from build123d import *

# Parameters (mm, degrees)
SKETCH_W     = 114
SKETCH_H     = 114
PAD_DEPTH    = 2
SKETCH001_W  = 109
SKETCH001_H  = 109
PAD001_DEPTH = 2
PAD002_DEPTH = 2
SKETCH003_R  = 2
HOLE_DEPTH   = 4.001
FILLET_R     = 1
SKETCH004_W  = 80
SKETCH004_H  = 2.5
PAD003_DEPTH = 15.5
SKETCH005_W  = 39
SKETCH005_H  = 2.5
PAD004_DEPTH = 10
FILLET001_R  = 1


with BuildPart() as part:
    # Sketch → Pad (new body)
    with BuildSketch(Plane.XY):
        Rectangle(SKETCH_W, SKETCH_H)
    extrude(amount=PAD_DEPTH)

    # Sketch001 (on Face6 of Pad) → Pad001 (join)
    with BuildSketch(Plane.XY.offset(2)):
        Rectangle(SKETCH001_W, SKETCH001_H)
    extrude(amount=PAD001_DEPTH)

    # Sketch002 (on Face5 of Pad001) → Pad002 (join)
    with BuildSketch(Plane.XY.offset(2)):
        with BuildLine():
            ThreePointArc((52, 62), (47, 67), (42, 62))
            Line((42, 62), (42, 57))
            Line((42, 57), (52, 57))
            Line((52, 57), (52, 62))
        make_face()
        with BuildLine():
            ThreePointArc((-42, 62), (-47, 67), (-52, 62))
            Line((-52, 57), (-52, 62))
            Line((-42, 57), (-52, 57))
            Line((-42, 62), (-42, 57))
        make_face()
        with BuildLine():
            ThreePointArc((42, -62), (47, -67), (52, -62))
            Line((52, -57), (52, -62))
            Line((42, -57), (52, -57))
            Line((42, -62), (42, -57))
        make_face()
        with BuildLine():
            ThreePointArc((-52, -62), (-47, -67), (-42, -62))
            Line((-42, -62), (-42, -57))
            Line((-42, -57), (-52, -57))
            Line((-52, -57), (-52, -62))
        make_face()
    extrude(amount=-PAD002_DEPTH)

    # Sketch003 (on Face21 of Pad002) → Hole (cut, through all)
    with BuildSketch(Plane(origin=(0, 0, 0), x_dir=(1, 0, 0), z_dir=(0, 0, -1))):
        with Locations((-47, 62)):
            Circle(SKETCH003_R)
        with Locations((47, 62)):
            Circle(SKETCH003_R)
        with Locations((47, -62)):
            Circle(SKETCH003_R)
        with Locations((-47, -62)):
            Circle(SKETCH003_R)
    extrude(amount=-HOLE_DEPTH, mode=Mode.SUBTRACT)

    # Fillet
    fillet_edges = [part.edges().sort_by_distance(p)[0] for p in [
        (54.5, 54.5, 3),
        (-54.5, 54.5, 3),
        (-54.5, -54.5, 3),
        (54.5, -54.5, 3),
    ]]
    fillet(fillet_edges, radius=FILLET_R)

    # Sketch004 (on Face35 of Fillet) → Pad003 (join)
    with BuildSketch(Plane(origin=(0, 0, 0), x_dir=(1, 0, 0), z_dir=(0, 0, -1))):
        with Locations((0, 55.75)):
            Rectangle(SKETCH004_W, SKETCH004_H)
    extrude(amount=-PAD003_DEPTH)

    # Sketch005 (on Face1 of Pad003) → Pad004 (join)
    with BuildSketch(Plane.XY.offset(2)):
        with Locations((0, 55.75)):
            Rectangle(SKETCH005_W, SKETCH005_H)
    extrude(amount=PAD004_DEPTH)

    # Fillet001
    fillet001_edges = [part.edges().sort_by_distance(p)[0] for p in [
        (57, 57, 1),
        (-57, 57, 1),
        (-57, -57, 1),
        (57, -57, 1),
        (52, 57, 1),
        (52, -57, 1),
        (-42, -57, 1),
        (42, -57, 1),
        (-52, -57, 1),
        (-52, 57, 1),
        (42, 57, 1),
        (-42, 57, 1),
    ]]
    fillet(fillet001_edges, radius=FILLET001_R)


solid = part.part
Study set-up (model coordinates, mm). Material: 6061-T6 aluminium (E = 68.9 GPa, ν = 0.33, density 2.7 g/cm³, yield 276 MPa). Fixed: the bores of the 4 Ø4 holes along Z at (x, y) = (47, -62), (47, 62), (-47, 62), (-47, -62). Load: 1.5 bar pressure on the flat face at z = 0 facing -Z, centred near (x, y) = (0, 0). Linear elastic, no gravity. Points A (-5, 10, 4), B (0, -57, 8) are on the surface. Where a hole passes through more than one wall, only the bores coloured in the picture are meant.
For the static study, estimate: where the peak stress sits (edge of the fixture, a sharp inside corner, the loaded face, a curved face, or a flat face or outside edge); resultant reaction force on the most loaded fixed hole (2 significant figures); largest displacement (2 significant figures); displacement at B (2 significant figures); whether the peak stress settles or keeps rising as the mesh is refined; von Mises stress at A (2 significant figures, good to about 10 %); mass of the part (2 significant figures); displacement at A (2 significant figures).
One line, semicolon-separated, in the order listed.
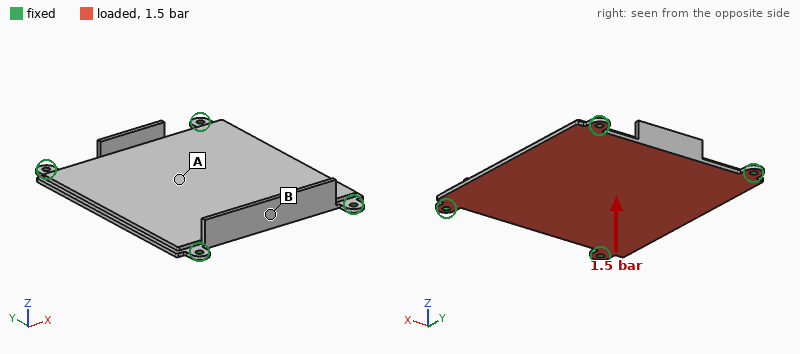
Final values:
edge of the fixture; 1.6 kN; 0.78 mm; 0.15 mm; keeps rising; 63 MPa; 150 g; 0.77 mm
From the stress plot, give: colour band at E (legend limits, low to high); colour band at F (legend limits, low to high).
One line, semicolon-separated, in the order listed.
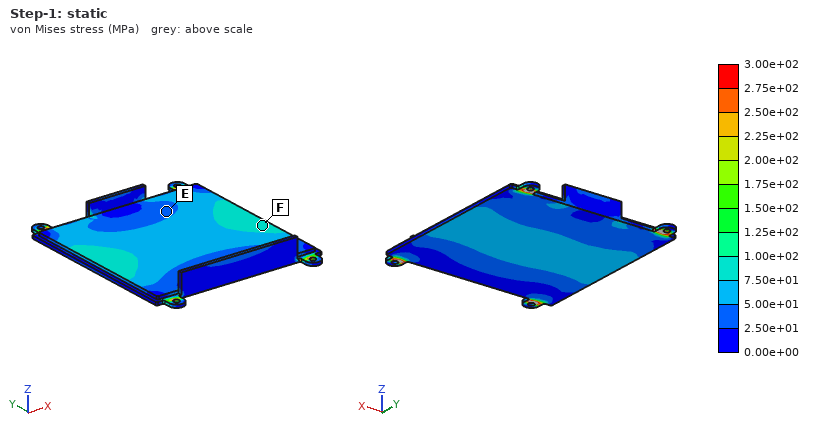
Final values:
2.50e+01 to 5.00e+01 MPa; 7.50e+01 to 1.00e+02 MPa
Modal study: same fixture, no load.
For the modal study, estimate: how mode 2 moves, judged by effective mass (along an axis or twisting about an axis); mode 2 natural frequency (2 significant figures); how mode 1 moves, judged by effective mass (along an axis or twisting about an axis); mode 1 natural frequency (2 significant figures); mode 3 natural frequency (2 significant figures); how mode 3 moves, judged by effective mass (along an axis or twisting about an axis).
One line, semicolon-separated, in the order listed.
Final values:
twisting about Y; 1200 Hz; along Z; 760 Hz; 1800 Hz; twisting about X
